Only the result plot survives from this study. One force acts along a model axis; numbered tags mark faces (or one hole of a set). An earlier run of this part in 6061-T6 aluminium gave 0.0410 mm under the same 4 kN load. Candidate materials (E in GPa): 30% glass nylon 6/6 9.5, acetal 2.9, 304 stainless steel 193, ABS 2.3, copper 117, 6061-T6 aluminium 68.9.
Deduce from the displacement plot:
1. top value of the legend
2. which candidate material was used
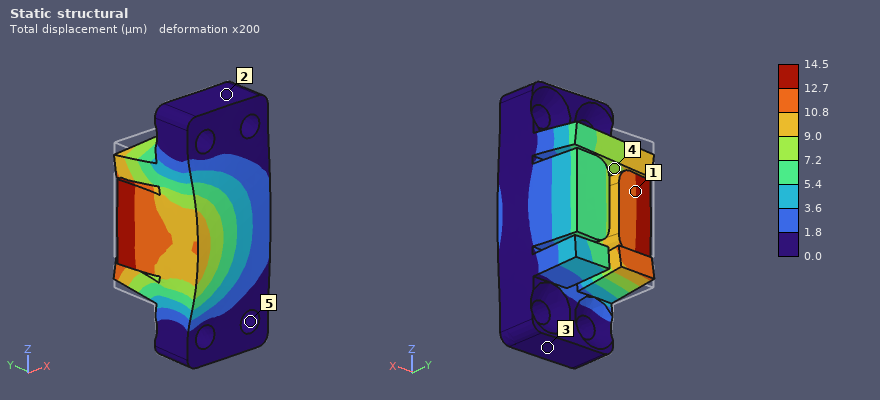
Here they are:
14.5 µm
304 stainless steel
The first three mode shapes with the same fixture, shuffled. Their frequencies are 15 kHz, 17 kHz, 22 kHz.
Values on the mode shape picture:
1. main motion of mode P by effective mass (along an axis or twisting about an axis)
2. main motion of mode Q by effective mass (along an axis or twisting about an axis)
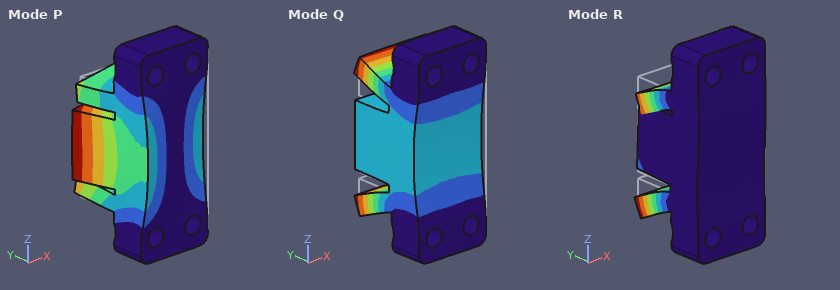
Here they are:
along X
along Y
